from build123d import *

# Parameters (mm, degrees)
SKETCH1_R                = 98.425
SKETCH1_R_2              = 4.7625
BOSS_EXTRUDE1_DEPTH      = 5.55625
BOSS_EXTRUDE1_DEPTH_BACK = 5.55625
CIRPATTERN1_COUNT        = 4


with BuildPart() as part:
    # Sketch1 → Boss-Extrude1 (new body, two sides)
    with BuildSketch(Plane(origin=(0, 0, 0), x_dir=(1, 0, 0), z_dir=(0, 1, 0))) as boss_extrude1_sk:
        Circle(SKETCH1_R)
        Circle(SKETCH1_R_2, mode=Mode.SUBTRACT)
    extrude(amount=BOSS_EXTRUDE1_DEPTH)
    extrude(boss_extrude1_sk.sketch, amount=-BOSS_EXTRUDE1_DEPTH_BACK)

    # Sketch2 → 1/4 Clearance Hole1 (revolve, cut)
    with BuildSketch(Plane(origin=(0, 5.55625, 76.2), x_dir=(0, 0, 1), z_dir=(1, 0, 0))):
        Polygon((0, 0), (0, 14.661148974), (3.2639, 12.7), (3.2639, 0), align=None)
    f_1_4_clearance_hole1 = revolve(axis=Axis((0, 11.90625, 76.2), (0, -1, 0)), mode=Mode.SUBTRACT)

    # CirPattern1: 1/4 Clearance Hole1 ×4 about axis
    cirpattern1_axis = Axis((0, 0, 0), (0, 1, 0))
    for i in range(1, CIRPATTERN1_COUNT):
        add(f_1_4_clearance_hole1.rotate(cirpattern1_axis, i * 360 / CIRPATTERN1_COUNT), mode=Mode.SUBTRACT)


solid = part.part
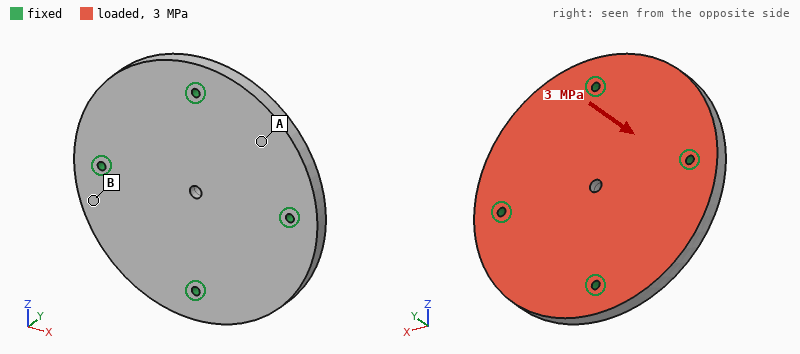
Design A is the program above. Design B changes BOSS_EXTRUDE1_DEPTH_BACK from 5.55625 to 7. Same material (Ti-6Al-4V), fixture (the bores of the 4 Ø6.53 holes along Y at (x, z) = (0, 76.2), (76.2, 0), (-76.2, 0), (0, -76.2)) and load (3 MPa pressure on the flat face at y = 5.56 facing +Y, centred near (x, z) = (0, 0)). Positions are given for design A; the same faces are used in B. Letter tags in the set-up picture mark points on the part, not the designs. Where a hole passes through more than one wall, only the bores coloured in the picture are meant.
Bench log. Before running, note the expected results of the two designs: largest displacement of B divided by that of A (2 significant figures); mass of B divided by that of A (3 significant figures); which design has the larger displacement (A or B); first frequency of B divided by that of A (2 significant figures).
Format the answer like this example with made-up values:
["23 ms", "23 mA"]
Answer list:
["0.73", "1.13", "A", "1.1"]
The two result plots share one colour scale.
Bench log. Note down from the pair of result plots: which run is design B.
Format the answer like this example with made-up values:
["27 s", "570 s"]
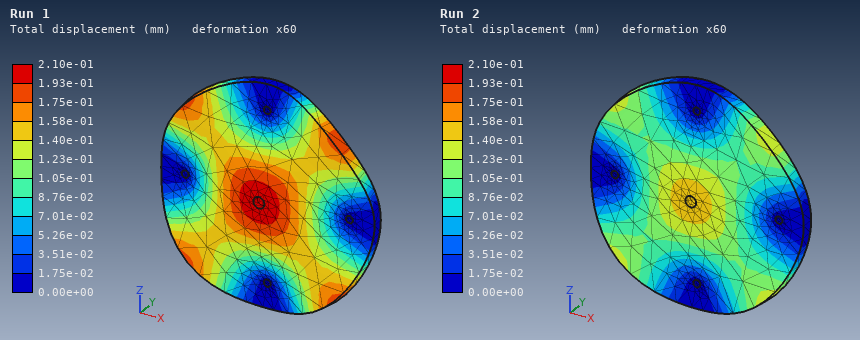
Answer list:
["Run 2"]
